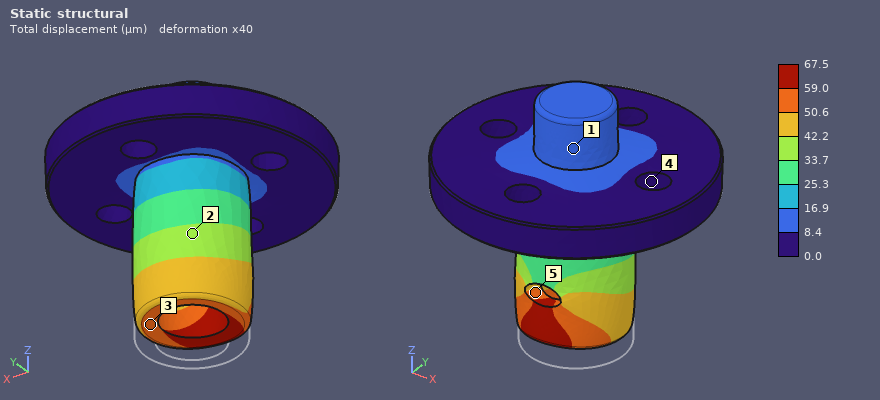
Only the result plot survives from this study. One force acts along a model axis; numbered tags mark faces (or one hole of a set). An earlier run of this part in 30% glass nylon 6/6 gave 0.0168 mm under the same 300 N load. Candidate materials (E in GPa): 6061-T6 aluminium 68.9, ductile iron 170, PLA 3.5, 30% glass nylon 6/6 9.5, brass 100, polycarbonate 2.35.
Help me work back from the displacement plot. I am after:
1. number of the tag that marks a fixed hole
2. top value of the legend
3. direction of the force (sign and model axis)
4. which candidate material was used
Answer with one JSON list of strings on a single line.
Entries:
["4", "67.5 µm", "+Z", "polycarbonate"]
